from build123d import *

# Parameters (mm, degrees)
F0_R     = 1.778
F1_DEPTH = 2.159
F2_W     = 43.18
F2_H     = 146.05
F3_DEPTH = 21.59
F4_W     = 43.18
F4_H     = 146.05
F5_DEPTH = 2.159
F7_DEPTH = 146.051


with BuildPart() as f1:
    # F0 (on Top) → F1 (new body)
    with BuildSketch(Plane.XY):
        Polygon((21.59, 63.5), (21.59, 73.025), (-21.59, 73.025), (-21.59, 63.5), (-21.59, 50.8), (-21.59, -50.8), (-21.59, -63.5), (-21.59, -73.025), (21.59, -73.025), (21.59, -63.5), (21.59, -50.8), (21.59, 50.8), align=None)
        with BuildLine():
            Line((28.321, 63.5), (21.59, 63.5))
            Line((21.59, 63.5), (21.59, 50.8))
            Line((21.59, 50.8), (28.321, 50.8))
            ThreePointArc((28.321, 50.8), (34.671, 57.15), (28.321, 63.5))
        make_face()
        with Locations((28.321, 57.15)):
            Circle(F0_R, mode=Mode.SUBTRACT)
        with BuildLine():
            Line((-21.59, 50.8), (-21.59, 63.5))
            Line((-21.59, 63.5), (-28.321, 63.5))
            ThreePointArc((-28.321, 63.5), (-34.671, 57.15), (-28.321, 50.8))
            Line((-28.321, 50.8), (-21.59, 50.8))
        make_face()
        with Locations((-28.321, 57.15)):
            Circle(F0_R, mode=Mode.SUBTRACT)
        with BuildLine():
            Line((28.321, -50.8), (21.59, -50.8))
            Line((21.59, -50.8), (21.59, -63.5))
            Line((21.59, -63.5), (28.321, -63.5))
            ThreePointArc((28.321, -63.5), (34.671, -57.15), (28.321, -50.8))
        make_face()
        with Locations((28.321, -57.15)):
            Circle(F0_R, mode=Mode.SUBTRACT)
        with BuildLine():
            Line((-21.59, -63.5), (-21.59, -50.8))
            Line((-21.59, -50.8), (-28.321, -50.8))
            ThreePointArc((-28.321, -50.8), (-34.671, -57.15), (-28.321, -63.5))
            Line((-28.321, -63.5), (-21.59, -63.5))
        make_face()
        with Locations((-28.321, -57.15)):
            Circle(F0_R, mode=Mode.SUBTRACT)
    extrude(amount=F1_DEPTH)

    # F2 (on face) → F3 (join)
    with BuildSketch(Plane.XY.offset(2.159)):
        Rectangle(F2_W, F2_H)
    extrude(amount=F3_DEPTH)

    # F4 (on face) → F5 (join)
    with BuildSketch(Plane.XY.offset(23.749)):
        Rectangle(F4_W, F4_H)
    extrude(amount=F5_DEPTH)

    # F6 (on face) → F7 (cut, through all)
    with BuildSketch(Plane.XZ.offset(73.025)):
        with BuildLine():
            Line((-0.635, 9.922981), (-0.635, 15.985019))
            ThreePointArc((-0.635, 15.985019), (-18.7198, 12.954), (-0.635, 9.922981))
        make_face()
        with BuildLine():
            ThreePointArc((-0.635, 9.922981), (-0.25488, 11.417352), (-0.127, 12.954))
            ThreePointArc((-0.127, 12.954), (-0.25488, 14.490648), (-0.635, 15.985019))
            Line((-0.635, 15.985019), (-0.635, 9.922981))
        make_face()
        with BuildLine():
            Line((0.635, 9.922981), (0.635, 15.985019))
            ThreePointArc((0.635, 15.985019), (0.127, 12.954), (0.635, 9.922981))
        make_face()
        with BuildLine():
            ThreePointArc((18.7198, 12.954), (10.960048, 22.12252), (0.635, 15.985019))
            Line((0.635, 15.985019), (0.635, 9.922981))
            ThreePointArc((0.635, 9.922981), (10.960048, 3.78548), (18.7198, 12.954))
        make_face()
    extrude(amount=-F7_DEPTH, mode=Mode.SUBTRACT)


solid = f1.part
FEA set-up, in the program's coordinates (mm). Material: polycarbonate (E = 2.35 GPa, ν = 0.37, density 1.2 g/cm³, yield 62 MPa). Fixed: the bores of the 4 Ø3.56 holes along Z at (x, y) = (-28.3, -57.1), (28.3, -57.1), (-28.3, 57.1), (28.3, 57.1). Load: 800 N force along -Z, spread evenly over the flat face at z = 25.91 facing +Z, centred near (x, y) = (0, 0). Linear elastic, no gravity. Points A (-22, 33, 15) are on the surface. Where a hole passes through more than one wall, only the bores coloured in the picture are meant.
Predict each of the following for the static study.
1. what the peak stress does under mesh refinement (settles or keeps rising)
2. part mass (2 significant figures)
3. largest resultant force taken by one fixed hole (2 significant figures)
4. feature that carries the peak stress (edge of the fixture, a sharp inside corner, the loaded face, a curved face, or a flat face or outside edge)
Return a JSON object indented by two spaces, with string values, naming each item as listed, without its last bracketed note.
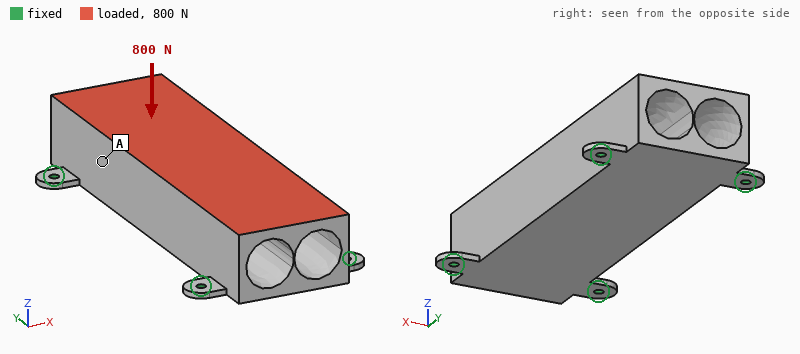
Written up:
{
  "what the peak stress does under mesh refinement": "keeps rising",
  "part mass": "100 g",
  "largest resultant force taken by one fixed hole": "220 N",
  "feature that carries the peak stress": "edge of the fixture"
}
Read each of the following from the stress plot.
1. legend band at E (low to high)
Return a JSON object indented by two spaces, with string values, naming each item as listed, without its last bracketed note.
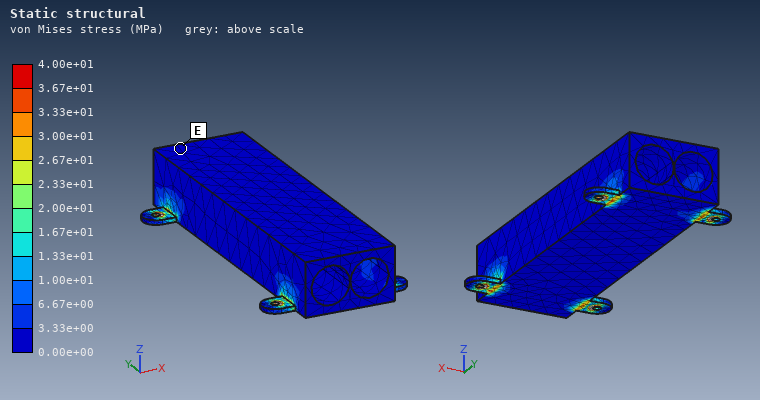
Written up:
{
  "legend band at E": "0.00e+00 to 3.33e+00 MPa"
}
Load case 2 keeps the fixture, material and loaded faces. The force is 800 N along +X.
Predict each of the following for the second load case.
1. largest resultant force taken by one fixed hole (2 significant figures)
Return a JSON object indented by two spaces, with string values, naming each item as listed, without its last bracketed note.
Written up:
{
  "largest resultant force taken by one fixed hole": "290 N"
}
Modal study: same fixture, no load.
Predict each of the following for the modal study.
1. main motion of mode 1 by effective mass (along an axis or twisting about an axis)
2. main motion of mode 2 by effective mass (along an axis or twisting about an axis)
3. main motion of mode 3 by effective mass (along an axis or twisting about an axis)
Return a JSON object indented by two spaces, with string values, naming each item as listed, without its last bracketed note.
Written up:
{
  "main motion of mode 1 by effective mass": "along Z",
  "main motion of mode 2 by effective mass": "along X",
  "main motion of mode 3 by effective mass": "along Y"
}
